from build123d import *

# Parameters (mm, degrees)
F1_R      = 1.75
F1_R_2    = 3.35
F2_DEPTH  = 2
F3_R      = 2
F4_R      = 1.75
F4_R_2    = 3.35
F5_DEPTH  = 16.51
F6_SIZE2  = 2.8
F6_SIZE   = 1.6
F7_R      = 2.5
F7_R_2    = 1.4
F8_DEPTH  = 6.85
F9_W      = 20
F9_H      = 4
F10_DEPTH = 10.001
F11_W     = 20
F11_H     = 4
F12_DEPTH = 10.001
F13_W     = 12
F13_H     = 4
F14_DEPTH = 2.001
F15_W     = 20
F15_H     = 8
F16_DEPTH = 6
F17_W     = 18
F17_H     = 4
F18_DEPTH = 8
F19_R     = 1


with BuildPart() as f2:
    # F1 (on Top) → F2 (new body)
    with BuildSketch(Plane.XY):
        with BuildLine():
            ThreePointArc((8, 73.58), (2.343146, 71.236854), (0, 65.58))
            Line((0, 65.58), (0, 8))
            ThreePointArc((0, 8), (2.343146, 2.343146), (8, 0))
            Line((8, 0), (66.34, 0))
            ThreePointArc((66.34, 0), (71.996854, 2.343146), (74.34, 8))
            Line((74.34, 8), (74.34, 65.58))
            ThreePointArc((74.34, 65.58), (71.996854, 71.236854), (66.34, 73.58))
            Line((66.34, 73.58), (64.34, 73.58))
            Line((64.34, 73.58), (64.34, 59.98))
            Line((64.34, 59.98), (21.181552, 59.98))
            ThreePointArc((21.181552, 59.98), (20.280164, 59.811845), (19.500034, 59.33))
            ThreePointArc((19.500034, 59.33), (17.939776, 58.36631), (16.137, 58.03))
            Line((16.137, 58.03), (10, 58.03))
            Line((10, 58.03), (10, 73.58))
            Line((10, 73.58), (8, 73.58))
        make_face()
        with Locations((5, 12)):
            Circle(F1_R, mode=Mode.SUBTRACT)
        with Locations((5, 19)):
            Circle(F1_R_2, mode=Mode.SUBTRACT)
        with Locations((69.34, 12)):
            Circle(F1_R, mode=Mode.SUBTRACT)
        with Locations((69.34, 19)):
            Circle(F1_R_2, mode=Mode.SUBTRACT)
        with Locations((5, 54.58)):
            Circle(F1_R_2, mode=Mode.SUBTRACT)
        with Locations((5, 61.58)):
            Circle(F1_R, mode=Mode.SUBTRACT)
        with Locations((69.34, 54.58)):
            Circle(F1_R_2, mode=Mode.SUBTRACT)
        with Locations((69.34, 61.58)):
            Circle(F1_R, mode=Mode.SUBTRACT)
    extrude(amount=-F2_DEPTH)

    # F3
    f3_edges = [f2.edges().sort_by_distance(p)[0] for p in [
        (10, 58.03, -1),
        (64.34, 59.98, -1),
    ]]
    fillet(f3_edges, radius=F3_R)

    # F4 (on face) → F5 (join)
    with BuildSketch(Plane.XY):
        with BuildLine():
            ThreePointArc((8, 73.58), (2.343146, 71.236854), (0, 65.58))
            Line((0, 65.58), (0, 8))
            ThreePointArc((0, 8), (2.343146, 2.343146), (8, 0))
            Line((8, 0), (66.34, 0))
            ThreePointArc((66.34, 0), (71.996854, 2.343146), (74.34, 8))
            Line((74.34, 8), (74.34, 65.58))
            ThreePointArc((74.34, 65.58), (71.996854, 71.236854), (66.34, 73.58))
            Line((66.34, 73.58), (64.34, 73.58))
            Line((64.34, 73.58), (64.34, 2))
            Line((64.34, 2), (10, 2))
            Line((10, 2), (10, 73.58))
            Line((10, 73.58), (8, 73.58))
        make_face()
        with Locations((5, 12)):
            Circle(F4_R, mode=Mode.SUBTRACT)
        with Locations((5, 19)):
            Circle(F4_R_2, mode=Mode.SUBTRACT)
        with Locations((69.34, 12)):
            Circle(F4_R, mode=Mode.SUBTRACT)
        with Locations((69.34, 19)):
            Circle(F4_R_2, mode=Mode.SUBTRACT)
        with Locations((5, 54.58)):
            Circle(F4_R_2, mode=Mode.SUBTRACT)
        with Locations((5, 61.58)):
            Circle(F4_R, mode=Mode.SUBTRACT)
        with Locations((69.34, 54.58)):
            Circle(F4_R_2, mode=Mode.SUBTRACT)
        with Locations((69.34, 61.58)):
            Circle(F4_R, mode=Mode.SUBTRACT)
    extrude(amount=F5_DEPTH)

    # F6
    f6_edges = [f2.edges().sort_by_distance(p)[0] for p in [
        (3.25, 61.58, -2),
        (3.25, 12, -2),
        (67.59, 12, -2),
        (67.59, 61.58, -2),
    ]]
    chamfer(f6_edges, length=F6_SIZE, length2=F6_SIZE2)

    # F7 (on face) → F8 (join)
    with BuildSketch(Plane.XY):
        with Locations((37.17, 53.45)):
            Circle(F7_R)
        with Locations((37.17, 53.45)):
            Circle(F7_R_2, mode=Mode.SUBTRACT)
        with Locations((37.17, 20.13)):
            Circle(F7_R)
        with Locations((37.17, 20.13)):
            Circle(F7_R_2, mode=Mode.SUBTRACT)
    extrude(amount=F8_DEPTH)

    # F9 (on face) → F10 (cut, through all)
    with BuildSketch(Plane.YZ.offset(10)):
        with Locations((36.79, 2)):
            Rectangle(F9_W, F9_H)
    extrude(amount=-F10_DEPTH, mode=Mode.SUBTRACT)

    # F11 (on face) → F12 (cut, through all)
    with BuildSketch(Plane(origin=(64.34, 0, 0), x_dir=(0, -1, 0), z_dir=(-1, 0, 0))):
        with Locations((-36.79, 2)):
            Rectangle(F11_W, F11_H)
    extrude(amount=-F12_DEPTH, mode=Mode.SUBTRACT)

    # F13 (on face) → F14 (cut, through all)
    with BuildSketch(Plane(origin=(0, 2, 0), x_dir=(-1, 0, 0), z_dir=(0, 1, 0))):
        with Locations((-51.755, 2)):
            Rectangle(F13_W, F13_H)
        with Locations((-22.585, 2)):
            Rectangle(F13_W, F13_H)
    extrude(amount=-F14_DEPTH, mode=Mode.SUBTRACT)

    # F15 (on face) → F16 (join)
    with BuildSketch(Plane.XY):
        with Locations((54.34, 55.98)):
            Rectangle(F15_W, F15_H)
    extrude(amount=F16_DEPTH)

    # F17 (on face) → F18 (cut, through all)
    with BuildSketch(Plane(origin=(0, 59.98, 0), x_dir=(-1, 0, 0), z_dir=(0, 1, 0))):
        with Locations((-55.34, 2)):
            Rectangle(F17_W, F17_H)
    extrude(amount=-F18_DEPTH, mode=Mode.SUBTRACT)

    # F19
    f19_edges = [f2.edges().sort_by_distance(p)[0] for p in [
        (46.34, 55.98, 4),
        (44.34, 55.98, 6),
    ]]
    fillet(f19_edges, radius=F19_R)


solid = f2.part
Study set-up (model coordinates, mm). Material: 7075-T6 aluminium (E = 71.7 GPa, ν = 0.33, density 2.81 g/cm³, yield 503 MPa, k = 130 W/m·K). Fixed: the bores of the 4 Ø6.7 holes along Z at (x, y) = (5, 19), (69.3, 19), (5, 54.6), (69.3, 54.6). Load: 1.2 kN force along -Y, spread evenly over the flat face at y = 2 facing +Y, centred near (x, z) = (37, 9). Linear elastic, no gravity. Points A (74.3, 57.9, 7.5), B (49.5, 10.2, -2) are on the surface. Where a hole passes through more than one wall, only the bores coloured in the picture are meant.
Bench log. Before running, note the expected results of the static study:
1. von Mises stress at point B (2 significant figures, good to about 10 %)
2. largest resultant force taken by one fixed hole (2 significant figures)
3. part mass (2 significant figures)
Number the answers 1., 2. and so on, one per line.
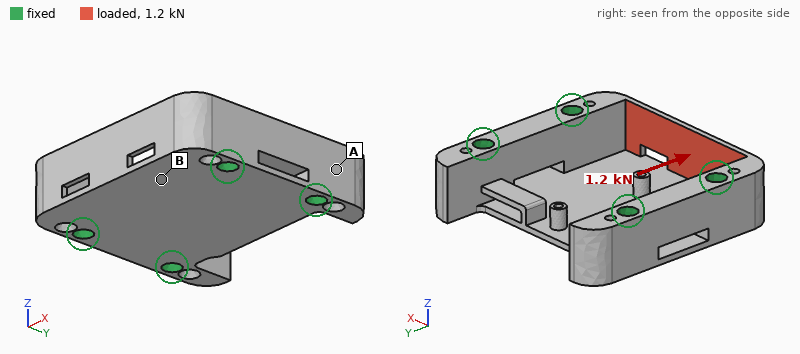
1. 32 MPa
2. 530 N
3. 84 g
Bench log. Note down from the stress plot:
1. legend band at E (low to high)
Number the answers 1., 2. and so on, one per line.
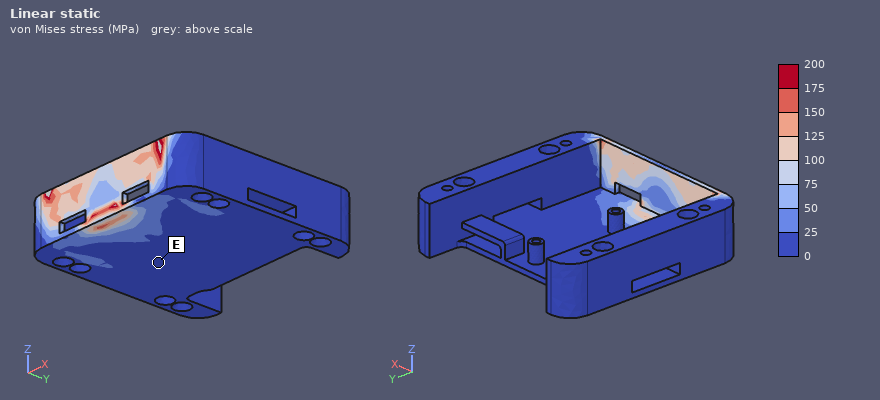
1. 0 to 25 MPa
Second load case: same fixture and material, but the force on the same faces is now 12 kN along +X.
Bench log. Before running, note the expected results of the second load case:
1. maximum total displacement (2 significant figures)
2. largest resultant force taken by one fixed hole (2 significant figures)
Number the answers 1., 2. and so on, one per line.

1. 0.10 mm
2. 6.0 kN
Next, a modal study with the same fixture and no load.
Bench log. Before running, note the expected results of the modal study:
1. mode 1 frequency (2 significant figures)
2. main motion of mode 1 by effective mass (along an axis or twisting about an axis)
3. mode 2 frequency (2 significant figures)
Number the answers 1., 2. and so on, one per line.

1. 3600 Hz
2. along Z
3. 5000 Hz
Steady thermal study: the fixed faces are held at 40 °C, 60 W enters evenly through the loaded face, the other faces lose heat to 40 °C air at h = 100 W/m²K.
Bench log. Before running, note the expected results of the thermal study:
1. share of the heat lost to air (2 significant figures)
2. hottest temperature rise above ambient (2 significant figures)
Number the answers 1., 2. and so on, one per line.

1. 23 %
2. 73 K
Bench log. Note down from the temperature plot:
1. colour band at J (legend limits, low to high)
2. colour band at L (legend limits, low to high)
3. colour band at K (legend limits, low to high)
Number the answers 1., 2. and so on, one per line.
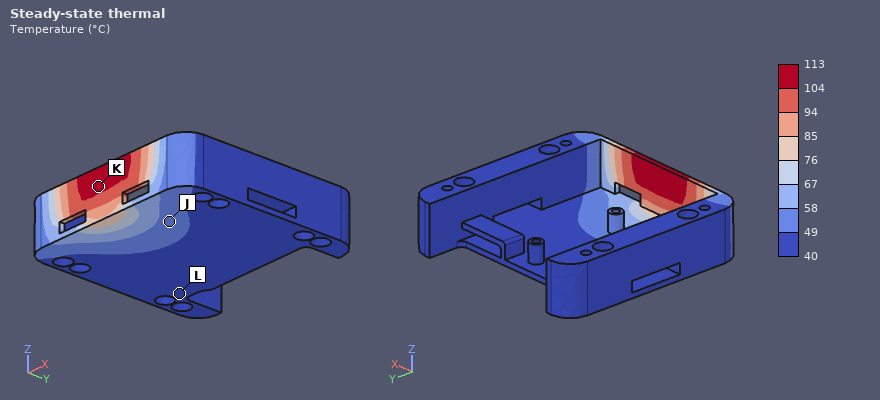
1. 49 to 58 °C
2. 40 to 49 °C
3. 104 to 113 °C
